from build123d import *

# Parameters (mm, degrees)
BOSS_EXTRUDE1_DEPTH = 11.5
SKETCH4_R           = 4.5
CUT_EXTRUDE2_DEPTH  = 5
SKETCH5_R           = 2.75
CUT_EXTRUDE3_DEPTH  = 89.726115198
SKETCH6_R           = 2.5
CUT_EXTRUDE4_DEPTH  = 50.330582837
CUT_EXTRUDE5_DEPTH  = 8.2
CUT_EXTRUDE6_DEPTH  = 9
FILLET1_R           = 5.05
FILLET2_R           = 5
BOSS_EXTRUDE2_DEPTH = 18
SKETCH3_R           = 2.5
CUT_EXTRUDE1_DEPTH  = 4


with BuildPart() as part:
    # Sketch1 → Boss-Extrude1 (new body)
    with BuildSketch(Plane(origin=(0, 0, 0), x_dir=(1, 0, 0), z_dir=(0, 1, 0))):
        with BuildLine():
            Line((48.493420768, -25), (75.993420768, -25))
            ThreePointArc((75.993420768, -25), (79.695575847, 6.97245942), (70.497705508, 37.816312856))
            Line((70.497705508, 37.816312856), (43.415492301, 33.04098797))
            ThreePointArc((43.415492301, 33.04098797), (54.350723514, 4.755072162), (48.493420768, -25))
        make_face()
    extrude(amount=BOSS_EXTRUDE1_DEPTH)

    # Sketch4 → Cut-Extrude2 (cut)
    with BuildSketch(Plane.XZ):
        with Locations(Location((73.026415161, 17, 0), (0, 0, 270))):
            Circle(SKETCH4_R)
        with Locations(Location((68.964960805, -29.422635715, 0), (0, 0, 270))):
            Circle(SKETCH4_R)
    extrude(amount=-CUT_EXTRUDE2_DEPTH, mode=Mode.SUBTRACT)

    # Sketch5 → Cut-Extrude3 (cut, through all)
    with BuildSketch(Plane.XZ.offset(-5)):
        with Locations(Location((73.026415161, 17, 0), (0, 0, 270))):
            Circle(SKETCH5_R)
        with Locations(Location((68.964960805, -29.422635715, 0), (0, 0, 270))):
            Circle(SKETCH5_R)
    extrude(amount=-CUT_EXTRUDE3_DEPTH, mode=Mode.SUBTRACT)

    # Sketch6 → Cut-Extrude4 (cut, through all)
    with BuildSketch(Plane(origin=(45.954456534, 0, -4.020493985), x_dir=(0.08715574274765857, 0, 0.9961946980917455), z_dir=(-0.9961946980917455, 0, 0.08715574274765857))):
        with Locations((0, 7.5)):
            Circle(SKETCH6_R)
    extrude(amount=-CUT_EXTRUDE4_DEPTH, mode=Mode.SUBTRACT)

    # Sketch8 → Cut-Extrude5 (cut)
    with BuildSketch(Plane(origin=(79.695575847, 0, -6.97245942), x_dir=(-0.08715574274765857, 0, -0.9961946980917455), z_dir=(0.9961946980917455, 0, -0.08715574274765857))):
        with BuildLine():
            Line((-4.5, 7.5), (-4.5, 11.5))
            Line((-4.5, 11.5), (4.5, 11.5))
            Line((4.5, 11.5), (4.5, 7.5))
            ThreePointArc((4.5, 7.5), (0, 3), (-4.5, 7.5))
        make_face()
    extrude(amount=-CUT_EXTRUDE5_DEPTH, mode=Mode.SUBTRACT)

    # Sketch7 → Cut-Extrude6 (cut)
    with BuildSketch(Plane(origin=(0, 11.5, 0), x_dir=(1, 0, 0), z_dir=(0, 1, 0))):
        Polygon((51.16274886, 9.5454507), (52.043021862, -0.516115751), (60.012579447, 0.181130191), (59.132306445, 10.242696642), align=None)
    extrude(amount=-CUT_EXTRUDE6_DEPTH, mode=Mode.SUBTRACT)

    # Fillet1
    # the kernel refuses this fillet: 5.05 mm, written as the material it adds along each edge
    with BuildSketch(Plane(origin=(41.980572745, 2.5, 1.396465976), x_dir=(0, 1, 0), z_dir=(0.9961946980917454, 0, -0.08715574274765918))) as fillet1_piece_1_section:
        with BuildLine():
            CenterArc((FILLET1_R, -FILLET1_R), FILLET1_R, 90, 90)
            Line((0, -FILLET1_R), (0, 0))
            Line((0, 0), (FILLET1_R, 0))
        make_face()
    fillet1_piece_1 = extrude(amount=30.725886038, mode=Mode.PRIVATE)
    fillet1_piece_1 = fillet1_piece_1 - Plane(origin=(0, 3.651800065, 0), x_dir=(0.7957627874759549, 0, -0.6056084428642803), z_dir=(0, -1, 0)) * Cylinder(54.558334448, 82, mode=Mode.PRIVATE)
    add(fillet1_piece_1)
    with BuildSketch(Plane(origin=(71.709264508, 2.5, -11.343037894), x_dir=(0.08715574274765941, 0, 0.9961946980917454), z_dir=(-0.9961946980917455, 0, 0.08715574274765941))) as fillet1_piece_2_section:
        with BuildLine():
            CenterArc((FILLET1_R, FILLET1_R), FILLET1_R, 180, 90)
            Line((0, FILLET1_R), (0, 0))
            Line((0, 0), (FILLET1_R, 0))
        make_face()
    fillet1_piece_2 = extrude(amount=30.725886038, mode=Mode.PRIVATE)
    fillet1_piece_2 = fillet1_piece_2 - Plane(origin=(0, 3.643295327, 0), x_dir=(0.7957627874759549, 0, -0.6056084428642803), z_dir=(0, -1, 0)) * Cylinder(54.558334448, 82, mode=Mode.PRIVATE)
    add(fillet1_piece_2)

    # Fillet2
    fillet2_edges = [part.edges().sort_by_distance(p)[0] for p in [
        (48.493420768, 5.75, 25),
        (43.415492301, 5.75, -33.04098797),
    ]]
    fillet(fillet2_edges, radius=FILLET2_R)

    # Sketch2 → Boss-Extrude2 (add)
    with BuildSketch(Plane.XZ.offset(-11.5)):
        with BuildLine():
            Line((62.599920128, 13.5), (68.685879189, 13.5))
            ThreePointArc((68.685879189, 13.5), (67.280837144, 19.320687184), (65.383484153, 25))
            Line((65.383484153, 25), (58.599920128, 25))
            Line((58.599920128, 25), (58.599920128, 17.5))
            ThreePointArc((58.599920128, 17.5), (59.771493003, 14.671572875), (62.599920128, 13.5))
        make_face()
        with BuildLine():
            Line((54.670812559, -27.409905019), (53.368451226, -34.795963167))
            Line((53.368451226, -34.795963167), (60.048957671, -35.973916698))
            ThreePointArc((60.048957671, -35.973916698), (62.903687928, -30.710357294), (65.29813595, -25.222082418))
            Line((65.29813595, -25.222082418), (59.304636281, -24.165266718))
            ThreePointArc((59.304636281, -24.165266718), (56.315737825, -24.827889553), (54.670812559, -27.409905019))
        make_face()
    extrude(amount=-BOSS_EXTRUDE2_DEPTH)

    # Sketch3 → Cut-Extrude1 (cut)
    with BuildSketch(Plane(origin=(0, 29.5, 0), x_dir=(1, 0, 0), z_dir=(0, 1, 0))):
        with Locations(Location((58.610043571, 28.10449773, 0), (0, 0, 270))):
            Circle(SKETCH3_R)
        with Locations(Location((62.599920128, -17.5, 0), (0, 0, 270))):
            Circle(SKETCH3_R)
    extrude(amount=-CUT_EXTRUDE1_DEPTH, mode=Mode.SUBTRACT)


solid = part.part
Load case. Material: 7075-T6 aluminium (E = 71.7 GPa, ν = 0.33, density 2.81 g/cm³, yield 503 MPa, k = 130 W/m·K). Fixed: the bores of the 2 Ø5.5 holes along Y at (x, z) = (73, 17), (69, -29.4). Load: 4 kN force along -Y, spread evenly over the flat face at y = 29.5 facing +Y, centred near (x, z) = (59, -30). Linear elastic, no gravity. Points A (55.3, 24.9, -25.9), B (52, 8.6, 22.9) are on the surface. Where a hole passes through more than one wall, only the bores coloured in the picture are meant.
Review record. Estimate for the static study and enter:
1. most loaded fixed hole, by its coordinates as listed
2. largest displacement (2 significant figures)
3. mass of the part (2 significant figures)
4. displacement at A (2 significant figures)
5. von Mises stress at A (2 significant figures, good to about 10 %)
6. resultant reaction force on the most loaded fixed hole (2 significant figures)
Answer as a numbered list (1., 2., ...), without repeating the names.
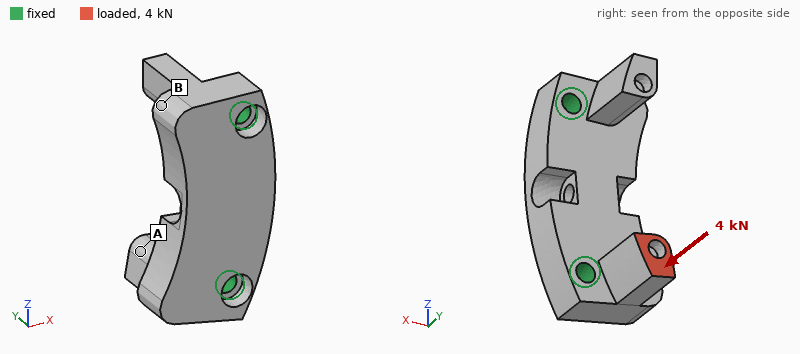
1. (69, -29.4)
2. 96 µm
3. 54 g
4. 74 µm
5. 44 MPa
6. 4.0 kN
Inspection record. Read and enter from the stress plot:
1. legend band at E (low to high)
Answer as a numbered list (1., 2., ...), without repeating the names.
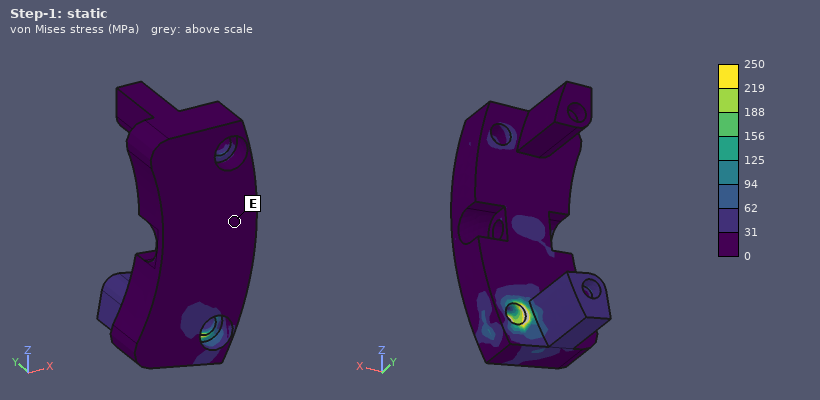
1. 0 to 31 MPa
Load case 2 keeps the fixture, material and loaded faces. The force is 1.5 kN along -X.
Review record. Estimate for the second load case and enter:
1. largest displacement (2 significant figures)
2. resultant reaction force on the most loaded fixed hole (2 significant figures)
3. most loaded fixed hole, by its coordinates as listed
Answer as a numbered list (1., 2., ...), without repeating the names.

1. 0.20 mm
2. 1.6 kN
3. (69, -29.4)
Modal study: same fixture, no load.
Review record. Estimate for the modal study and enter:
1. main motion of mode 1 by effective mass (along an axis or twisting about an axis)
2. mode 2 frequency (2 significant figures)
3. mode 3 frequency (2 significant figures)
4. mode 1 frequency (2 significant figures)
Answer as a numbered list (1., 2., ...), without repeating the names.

1. along Y
2. 10 kHz
3. 12 kHz
4. 7700 Hz
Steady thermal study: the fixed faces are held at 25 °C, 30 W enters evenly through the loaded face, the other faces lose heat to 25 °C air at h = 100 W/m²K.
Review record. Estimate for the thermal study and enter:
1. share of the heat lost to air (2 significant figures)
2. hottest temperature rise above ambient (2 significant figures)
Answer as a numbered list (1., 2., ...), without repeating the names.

1. 15 %
2. 58 K
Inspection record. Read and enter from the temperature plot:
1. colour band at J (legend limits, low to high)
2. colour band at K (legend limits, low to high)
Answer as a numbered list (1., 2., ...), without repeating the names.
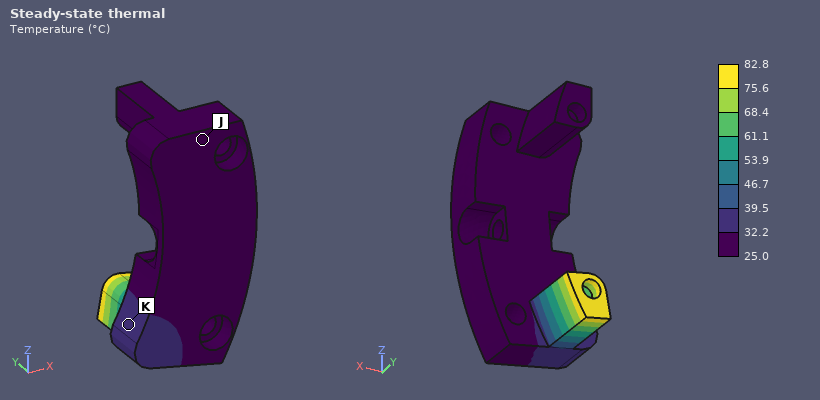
1. 25.0 to 32.2 °C
2. 32.2 to 39.5 °C
